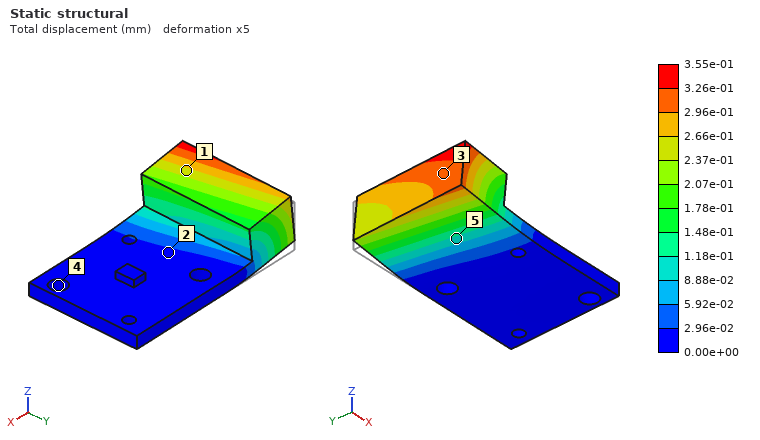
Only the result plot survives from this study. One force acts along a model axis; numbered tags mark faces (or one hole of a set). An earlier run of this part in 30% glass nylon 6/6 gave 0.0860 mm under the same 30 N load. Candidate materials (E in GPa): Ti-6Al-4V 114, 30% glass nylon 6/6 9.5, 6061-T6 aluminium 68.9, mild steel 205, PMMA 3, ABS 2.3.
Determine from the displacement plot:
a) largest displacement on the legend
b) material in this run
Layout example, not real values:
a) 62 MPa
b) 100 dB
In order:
a) 3.55e-01 mm
b) ABS
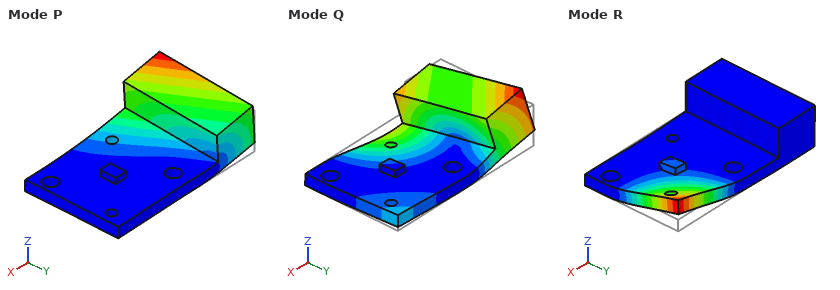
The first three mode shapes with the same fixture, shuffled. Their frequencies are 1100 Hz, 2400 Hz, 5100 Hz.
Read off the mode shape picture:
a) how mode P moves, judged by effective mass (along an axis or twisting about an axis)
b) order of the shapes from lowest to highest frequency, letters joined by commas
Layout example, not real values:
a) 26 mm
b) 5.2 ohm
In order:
a) along Z
b) P, Q, R
